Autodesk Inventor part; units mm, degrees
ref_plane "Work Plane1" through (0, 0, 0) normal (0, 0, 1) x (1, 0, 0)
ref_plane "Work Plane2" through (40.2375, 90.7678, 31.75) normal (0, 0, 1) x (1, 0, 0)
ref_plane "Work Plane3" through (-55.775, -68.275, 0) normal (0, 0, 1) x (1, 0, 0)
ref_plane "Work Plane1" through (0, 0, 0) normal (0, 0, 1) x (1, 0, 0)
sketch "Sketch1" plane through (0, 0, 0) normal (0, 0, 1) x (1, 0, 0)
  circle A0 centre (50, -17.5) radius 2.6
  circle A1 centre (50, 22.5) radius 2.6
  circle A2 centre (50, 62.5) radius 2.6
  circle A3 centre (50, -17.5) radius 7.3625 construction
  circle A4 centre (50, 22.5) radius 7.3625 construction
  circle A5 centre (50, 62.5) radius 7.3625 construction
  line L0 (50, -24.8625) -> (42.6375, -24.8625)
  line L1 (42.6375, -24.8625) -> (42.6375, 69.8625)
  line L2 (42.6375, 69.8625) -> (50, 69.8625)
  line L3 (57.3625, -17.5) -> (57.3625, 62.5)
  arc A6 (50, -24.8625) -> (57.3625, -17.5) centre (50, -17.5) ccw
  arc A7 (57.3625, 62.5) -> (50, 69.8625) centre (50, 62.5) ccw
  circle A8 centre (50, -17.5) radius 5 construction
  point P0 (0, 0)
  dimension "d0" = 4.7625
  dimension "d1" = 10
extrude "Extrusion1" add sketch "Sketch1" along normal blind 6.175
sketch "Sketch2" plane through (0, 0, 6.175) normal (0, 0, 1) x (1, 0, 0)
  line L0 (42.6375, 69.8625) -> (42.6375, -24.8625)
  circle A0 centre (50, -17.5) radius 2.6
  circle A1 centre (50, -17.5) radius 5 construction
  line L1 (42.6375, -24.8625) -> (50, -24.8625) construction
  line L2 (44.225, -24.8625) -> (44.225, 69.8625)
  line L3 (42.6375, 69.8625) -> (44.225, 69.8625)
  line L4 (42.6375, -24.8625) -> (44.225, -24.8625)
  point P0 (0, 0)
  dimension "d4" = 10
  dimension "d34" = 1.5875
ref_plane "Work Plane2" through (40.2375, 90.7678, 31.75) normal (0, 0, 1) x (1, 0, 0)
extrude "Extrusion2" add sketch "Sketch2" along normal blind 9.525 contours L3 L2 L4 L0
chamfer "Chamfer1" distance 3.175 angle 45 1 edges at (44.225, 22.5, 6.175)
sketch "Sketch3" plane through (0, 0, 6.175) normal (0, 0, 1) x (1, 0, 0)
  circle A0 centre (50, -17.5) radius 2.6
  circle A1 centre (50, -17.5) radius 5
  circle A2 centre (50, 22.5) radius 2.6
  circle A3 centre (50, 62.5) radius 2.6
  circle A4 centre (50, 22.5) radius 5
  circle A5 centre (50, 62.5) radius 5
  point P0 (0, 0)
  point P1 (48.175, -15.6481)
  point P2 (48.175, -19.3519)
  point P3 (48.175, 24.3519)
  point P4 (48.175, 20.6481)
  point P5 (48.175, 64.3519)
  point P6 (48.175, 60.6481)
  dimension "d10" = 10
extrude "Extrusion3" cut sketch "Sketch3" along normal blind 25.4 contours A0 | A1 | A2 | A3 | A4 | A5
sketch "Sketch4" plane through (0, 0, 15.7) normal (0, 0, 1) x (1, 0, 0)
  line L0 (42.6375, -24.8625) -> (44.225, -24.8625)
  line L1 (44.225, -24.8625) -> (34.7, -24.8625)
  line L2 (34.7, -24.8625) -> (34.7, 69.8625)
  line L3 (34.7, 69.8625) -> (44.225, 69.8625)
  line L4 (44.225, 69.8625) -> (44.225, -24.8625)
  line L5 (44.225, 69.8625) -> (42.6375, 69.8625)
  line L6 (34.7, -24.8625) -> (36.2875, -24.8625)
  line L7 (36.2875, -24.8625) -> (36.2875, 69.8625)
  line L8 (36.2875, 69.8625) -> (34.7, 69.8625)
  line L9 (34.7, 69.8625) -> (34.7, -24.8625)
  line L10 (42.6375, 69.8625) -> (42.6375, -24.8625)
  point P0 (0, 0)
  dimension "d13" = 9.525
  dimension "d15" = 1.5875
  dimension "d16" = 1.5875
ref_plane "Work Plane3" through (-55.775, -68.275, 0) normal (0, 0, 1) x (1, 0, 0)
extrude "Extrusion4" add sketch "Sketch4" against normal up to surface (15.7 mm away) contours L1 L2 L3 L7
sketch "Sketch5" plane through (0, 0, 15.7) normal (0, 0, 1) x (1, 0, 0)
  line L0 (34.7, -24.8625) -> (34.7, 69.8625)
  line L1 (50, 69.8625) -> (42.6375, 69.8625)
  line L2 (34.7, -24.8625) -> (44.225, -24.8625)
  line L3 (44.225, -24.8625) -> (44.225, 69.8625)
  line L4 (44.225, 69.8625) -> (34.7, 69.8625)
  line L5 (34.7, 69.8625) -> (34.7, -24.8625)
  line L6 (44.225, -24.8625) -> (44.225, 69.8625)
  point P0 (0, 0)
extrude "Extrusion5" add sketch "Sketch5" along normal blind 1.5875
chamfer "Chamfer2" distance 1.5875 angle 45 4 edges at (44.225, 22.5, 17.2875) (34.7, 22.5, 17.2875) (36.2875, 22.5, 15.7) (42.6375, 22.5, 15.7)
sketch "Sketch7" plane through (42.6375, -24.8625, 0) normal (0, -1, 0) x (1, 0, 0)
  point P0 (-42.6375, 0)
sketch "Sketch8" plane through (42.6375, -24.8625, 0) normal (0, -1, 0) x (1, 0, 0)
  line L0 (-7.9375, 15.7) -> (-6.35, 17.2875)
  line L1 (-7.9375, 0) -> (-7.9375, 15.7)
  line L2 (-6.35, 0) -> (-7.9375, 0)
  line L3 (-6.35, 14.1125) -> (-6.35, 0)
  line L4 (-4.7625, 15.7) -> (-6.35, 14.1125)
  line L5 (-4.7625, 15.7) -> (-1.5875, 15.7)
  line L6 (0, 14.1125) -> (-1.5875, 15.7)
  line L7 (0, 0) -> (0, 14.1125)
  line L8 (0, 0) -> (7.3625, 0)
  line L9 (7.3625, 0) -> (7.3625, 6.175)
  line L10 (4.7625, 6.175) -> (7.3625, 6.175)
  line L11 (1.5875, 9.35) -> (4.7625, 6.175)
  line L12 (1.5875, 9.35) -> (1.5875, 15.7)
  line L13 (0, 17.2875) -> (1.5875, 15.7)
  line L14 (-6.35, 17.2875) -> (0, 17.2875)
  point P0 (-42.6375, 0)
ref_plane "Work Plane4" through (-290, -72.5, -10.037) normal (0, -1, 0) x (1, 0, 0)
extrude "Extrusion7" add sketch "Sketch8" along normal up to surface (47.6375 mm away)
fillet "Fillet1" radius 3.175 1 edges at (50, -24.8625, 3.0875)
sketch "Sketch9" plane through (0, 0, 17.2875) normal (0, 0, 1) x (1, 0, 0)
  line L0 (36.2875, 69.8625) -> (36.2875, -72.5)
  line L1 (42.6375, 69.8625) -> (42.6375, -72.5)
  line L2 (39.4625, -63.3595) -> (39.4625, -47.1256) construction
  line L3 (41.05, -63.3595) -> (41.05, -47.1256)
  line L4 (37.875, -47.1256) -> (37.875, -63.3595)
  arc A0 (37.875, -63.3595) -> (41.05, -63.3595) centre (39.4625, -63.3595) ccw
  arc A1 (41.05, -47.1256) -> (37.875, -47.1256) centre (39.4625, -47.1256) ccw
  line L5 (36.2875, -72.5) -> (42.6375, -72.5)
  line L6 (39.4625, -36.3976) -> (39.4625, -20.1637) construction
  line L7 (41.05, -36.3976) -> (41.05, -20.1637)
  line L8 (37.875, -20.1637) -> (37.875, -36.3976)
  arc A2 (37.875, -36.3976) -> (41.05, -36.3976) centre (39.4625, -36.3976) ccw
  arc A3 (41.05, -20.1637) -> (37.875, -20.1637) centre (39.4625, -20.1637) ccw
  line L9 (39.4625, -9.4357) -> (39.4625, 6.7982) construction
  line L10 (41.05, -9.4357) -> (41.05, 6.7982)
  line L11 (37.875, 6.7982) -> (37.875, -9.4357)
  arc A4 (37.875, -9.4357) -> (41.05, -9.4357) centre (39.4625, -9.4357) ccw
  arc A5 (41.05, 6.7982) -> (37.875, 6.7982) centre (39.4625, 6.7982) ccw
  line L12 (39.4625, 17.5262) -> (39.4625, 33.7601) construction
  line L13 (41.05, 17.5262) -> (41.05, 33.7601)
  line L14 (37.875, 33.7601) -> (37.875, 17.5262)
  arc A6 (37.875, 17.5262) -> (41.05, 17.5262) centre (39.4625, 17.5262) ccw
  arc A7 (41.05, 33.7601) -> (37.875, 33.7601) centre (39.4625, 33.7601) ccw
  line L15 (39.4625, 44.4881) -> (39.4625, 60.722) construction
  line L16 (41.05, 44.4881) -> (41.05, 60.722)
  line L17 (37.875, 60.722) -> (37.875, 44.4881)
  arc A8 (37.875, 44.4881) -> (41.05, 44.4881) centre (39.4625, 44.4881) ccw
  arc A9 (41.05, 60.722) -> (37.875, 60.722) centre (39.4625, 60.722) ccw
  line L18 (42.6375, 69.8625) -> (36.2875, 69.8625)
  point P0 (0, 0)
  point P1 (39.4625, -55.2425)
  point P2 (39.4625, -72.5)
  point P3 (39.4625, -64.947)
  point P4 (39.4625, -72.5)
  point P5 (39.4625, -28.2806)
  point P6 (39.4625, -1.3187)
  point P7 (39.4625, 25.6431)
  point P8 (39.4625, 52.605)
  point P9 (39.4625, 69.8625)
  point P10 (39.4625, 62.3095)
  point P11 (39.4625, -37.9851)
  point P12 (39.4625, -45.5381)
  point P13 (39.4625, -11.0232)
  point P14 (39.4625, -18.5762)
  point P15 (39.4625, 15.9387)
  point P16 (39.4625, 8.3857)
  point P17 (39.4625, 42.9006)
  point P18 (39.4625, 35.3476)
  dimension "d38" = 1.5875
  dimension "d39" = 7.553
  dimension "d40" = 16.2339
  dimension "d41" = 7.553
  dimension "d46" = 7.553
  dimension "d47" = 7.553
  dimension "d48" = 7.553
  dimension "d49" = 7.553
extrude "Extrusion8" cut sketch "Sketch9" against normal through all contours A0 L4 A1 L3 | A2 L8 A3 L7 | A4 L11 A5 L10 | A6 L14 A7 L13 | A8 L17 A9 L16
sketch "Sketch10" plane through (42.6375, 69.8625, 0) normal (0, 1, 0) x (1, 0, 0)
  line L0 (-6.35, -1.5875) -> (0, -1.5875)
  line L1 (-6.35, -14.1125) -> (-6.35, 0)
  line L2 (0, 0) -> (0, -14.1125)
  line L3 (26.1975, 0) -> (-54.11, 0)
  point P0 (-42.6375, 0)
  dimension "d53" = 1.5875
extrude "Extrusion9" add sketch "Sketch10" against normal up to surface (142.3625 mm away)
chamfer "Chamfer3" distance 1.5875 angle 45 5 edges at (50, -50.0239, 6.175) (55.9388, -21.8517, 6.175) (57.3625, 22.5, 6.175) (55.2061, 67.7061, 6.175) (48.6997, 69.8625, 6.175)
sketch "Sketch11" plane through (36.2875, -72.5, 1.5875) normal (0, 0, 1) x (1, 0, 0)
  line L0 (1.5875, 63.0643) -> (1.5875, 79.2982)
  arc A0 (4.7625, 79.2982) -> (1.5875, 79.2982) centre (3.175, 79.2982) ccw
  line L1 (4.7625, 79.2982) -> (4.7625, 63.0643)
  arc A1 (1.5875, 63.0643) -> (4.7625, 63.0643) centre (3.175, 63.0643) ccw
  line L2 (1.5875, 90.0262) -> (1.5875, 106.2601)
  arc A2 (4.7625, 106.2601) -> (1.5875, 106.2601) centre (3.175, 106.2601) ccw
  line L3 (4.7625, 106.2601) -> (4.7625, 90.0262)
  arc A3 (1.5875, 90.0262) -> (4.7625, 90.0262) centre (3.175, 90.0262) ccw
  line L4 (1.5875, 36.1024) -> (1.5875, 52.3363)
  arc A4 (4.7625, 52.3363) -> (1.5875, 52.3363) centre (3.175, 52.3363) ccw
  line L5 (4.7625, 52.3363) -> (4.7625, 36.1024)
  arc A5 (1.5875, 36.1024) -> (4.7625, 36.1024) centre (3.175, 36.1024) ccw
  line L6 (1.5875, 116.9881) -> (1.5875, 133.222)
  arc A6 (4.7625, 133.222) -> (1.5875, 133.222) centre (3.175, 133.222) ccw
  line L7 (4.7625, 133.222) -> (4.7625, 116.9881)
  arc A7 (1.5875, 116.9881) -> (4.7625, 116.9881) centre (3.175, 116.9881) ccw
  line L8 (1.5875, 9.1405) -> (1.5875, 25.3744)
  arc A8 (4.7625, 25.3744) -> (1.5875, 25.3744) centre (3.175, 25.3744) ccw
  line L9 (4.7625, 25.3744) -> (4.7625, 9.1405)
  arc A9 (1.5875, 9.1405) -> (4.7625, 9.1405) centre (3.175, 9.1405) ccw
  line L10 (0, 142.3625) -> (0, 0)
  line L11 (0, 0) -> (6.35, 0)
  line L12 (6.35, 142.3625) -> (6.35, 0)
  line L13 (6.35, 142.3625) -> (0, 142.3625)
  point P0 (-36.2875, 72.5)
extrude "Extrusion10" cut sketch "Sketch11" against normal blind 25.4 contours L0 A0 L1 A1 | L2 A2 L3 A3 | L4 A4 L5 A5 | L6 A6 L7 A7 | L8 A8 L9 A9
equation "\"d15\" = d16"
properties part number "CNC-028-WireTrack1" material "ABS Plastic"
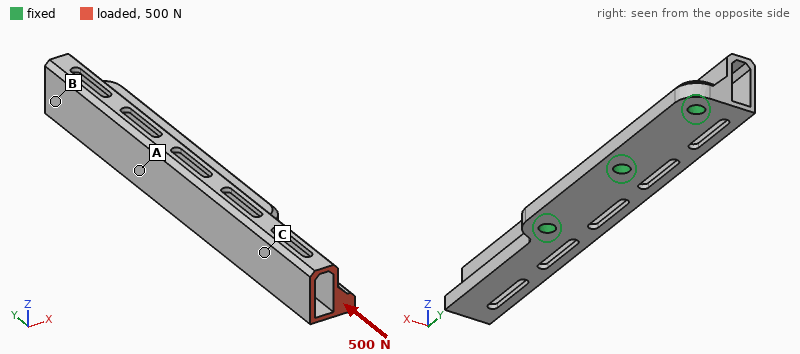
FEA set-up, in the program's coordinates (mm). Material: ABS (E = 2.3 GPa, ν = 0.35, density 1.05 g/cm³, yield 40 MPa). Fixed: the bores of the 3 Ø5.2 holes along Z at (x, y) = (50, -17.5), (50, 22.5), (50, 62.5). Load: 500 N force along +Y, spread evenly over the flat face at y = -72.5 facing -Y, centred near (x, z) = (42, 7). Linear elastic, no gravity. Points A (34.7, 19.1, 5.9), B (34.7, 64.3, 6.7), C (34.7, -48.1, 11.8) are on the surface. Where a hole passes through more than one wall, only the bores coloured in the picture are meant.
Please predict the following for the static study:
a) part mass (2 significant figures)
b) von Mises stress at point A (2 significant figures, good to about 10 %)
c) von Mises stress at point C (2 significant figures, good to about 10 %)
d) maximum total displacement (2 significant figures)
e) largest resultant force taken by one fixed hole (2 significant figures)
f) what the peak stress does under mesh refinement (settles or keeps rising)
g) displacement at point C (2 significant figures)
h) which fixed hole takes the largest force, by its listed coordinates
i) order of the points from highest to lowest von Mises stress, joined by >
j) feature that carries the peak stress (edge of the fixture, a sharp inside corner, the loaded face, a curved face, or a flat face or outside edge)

20 g
2.8 MPa
5.1 MPa
0.41 mm
340 N
keeps rising
0.25 mm
(50, -17.5)
C > A > B
edge of the fixture
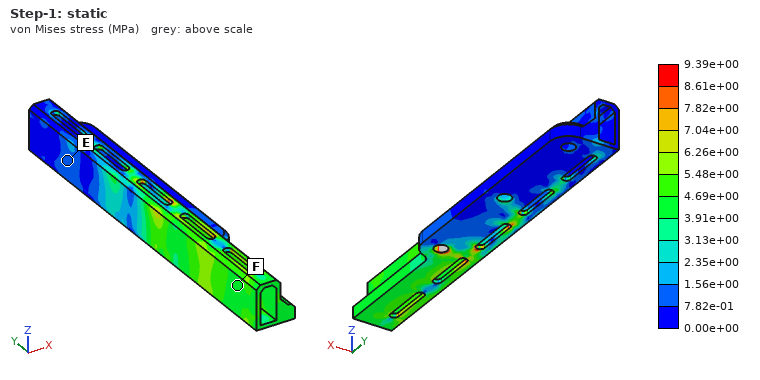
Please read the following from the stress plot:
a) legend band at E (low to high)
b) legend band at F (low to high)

7.82e-01 to 1.56e+00 MPa
3.91e+00 to 4.69e+00 MPa
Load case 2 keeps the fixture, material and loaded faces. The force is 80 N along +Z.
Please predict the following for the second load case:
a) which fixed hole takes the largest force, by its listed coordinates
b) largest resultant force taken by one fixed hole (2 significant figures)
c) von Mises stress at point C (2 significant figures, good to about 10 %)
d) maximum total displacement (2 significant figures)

(50, -17.5)
160 N
2.6 MPa
1.6 mm
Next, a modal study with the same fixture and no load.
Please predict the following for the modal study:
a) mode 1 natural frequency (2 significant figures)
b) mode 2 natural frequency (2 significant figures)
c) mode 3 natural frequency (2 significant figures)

710 Hz
1000 Hz
1500 Hz
